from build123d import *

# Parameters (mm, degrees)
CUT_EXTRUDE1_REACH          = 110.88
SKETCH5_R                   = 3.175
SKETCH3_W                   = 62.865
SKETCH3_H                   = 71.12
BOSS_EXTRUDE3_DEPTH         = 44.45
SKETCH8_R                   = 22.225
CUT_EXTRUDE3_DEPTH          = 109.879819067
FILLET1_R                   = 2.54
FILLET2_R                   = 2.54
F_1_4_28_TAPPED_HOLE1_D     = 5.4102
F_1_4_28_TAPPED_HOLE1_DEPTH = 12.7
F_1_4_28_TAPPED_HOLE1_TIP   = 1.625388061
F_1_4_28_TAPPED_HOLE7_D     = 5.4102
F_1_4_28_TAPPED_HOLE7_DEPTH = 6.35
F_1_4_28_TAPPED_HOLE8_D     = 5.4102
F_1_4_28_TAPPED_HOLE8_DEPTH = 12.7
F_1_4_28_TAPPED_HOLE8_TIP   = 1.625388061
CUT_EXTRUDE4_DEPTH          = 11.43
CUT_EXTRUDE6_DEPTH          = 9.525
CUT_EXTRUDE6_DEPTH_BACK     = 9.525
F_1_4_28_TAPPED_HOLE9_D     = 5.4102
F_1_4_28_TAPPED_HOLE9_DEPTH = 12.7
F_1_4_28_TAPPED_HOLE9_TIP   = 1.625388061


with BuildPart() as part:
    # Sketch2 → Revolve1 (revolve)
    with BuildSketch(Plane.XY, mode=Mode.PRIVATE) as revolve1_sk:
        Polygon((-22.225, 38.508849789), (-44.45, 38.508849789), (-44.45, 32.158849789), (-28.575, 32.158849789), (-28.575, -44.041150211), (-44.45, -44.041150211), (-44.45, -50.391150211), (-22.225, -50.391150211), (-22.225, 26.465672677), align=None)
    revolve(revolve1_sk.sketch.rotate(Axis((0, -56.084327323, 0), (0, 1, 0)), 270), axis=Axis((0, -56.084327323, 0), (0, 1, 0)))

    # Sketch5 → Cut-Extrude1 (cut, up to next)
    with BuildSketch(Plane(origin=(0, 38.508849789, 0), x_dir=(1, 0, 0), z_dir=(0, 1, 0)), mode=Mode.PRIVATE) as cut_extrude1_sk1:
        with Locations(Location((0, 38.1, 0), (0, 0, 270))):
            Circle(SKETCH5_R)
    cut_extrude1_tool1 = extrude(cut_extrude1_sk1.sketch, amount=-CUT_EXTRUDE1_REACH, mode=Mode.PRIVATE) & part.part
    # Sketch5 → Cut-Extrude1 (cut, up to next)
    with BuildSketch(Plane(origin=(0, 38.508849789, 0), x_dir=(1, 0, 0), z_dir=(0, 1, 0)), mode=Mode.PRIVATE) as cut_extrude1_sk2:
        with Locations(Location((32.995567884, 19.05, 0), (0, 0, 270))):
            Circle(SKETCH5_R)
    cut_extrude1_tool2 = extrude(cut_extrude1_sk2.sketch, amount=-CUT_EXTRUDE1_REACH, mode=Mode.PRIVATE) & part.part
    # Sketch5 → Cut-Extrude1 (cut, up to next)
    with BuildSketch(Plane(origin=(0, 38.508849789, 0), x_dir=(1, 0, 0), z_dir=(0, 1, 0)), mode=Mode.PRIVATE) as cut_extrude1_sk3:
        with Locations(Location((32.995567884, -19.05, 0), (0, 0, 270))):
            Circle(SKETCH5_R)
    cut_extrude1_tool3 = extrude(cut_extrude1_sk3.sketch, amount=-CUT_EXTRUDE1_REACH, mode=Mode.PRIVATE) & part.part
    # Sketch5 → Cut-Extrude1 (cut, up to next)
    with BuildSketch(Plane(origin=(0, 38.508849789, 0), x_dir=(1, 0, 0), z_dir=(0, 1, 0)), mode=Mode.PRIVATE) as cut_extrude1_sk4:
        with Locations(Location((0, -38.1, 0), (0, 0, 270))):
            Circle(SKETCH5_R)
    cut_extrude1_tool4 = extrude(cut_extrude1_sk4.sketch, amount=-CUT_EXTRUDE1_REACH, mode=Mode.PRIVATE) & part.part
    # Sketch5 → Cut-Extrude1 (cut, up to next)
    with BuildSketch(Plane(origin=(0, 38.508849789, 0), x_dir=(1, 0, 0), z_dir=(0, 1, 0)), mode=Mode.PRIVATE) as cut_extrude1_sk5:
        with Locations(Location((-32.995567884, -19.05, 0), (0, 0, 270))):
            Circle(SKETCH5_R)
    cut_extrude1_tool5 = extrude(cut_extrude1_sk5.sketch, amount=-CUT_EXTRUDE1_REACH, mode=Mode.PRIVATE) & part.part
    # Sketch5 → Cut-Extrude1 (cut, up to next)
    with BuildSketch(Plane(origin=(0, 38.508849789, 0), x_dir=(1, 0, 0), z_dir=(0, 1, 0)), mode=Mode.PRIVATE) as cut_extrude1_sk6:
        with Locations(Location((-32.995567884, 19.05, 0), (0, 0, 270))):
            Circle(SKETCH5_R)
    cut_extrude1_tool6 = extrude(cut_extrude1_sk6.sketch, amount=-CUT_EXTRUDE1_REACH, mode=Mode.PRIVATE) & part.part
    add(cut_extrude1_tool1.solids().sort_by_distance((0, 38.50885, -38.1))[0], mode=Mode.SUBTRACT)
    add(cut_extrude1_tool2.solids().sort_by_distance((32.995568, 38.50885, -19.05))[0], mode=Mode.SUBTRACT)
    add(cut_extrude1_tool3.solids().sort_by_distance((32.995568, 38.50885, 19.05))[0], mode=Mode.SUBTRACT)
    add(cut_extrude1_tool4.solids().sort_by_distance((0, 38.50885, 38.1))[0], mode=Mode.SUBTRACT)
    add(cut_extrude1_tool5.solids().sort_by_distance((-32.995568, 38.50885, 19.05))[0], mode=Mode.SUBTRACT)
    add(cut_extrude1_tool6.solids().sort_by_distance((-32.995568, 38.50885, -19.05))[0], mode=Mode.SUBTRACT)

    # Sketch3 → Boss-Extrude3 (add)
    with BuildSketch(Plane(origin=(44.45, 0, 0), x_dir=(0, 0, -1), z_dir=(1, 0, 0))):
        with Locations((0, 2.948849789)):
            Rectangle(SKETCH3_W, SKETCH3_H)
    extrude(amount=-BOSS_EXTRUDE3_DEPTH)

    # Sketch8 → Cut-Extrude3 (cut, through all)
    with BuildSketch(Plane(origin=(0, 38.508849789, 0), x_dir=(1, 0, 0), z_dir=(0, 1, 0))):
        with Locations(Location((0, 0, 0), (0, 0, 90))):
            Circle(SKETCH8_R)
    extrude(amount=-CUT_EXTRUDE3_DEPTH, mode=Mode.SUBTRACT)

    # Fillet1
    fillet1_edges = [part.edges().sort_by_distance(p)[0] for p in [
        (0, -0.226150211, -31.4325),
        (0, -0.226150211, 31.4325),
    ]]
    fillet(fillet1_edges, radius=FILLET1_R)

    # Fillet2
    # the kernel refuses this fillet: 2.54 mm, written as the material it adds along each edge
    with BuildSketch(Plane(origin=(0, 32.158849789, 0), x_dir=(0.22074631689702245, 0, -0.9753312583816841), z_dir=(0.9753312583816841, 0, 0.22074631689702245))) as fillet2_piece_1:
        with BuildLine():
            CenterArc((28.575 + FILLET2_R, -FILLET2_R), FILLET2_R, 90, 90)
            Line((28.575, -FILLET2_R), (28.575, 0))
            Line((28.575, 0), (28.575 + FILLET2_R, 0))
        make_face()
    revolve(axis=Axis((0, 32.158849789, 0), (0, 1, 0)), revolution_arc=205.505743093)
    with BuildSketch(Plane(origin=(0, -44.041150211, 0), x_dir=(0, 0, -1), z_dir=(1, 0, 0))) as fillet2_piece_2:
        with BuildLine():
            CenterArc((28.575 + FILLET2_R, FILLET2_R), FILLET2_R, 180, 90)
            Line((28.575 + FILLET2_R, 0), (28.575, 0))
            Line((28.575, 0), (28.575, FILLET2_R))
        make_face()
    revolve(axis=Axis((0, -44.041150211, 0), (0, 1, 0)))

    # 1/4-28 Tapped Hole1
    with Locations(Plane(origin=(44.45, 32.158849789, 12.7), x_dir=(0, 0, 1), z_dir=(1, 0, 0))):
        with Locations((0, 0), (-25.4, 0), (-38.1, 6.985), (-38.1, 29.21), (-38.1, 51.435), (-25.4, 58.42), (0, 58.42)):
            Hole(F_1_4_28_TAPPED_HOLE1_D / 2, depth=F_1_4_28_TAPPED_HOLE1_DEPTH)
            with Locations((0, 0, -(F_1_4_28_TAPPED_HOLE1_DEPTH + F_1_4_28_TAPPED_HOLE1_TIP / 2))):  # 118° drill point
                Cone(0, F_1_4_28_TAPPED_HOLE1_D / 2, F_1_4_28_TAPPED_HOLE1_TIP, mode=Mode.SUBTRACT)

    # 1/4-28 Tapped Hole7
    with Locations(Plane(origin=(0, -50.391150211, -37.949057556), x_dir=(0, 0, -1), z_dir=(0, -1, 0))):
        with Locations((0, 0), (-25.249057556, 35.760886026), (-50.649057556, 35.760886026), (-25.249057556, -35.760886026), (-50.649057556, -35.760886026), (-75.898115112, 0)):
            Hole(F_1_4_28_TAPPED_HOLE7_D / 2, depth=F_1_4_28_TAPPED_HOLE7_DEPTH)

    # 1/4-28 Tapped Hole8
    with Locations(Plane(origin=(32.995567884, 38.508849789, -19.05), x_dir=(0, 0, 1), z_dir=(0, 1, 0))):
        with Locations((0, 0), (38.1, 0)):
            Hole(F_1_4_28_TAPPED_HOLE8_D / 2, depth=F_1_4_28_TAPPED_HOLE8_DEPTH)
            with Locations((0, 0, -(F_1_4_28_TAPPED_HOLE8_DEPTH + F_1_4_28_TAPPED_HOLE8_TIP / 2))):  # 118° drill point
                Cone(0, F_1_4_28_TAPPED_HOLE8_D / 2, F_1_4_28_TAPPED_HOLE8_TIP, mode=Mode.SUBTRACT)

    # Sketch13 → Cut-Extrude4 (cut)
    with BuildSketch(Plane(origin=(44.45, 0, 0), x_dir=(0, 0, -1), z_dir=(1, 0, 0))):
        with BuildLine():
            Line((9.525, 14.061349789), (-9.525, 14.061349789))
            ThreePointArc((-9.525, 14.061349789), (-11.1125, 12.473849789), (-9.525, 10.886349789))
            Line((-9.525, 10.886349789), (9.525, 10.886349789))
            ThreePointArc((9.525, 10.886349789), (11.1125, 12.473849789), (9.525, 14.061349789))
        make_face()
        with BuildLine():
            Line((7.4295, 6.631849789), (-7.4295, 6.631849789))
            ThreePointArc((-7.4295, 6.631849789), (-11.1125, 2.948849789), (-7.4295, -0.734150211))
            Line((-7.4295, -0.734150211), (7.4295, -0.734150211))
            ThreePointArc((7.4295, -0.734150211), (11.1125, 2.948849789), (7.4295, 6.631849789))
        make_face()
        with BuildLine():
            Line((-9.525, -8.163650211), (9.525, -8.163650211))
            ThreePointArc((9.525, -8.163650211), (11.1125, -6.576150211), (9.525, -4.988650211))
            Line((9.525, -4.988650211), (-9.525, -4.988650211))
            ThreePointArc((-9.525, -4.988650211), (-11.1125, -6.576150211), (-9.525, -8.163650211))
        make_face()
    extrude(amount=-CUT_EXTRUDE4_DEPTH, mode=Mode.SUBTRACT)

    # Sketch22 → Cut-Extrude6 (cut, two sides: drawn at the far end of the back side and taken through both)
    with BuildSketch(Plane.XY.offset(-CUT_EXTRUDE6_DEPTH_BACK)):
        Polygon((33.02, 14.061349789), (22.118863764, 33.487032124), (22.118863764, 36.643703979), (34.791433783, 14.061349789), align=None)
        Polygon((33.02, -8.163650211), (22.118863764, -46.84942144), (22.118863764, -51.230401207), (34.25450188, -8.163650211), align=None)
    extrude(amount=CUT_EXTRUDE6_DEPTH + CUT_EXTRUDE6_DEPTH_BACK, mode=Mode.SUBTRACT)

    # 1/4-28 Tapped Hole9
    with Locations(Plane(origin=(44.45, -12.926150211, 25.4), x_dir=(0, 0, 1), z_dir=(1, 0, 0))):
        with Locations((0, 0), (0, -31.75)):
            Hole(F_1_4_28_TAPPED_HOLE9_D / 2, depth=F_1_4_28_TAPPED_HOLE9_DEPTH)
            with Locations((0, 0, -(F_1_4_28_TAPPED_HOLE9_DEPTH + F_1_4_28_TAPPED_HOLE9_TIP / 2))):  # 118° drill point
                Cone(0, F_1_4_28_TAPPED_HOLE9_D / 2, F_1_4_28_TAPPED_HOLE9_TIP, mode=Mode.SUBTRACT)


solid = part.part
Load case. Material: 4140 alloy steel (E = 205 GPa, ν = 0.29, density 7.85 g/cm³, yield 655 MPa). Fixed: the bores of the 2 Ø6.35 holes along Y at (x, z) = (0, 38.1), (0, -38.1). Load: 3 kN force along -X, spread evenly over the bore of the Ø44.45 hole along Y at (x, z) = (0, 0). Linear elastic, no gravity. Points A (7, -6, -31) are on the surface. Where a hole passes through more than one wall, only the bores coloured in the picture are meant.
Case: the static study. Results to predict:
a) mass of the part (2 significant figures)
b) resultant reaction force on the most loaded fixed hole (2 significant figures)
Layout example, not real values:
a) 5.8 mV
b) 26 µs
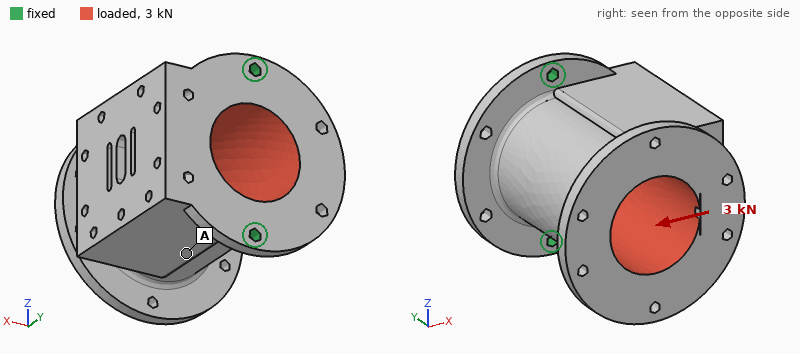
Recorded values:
a) 1.8 kg
b) 1.5 kN
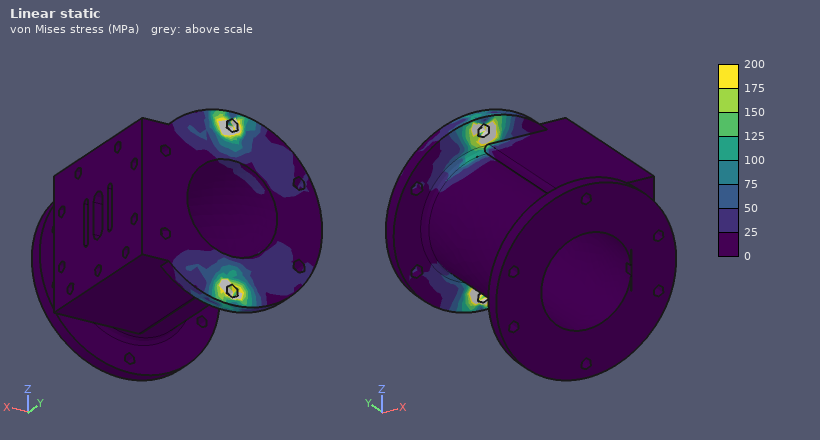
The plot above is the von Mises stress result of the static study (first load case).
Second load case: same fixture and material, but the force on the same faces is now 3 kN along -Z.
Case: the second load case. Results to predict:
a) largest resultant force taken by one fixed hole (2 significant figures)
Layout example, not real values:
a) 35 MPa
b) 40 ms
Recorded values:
a) 2.4 kN
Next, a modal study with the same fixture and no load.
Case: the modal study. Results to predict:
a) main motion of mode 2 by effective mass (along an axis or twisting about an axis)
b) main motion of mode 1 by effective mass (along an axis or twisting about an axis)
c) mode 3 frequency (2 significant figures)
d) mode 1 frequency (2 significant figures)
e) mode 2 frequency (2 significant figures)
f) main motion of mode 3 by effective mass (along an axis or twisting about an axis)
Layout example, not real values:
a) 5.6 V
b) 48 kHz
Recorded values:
a) along Z
b) along X
c) 3500 Hz
d) 480 Hz
e) 2100 Hz
f) along Y
